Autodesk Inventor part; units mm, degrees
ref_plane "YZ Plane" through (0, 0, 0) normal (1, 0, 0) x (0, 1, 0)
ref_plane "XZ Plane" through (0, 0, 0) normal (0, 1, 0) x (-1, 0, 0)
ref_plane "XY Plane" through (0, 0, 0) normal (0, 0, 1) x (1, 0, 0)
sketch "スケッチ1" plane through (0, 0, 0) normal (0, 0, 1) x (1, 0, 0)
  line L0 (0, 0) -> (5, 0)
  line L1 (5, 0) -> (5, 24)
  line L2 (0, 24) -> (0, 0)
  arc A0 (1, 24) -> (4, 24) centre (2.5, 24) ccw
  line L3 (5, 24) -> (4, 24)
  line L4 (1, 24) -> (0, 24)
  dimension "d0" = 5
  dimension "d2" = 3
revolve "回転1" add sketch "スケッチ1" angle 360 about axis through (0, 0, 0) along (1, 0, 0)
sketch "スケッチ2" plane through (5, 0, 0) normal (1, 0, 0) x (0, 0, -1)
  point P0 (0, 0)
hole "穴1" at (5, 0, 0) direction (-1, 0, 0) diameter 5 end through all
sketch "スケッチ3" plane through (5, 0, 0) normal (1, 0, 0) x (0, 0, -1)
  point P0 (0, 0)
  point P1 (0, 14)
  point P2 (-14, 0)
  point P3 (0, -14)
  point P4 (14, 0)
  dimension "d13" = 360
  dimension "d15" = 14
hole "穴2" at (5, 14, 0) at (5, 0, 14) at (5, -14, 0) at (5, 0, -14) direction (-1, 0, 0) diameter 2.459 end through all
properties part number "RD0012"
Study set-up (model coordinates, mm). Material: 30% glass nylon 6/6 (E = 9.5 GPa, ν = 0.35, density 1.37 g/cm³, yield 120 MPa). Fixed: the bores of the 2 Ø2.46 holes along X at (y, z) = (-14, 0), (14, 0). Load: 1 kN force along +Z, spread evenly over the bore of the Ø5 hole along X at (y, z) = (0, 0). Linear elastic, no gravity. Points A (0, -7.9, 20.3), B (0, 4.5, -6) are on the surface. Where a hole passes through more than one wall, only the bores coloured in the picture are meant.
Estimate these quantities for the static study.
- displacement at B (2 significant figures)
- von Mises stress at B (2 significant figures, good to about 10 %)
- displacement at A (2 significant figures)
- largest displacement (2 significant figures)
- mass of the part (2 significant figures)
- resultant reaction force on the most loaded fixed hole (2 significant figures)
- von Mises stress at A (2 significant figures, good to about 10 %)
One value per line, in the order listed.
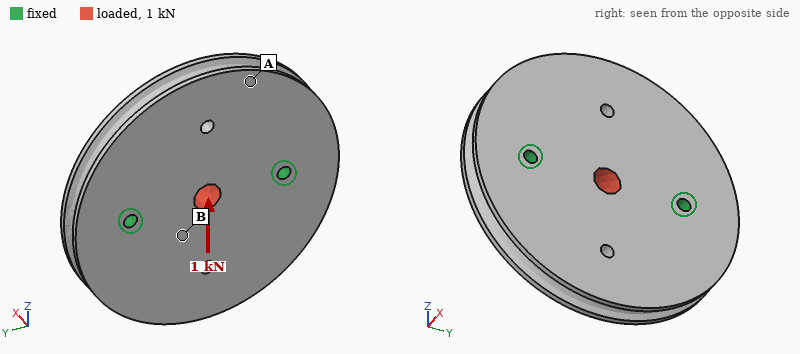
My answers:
13 µm
7.2 MPa
9.1 µm
20 µm
11 g
500 N
2.7 MPa
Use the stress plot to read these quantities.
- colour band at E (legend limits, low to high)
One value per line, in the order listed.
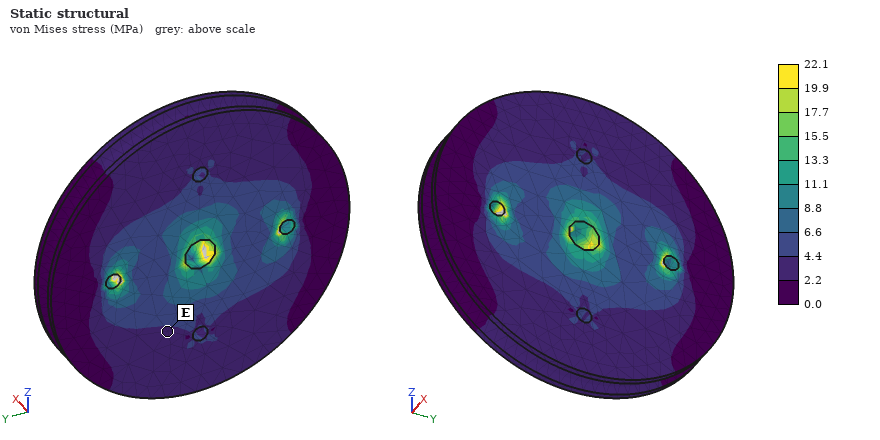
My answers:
2.2 to 4.4 MPa
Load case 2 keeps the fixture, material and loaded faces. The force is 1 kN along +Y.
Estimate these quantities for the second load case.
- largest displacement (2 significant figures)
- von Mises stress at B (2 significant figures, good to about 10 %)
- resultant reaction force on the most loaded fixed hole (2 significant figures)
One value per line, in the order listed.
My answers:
14 µm
2.9 MPa
500 N
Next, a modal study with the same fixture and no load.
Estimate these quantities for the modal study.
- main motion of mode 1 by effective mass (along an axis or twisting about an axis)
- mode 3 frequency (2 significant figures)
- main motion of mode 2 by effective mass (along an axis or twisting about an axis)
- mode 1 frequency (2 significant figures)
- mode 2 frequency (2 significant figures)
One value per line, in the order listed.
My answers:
twisting about Y
8000 Hz
along X
3400 Hz
4600 Hz
